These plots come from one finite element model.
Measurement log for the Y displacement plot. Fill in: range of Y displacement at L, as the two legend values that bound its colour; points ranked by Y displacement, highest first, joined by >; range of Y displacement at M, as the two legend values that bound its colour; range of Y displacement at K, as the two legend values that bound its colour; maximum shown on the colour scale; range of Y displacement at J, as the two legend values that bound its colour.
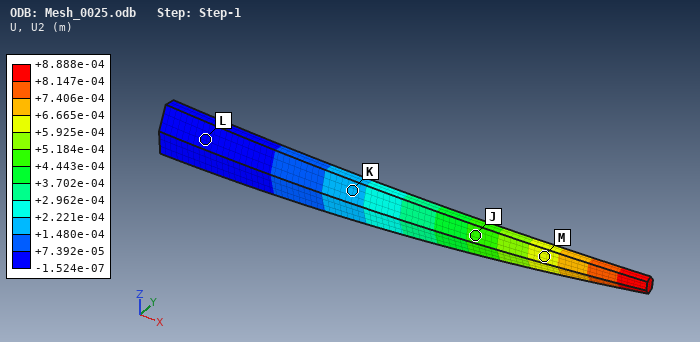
-1.524e-07 to +7.392e-05 m
M > J > K > L
+5.925e-04 to +6.665e-04 m
+1.480e-04 to +2.221e-04 m
+8.888e-04 m
+4.443e-04 to +5.184e-04 m
